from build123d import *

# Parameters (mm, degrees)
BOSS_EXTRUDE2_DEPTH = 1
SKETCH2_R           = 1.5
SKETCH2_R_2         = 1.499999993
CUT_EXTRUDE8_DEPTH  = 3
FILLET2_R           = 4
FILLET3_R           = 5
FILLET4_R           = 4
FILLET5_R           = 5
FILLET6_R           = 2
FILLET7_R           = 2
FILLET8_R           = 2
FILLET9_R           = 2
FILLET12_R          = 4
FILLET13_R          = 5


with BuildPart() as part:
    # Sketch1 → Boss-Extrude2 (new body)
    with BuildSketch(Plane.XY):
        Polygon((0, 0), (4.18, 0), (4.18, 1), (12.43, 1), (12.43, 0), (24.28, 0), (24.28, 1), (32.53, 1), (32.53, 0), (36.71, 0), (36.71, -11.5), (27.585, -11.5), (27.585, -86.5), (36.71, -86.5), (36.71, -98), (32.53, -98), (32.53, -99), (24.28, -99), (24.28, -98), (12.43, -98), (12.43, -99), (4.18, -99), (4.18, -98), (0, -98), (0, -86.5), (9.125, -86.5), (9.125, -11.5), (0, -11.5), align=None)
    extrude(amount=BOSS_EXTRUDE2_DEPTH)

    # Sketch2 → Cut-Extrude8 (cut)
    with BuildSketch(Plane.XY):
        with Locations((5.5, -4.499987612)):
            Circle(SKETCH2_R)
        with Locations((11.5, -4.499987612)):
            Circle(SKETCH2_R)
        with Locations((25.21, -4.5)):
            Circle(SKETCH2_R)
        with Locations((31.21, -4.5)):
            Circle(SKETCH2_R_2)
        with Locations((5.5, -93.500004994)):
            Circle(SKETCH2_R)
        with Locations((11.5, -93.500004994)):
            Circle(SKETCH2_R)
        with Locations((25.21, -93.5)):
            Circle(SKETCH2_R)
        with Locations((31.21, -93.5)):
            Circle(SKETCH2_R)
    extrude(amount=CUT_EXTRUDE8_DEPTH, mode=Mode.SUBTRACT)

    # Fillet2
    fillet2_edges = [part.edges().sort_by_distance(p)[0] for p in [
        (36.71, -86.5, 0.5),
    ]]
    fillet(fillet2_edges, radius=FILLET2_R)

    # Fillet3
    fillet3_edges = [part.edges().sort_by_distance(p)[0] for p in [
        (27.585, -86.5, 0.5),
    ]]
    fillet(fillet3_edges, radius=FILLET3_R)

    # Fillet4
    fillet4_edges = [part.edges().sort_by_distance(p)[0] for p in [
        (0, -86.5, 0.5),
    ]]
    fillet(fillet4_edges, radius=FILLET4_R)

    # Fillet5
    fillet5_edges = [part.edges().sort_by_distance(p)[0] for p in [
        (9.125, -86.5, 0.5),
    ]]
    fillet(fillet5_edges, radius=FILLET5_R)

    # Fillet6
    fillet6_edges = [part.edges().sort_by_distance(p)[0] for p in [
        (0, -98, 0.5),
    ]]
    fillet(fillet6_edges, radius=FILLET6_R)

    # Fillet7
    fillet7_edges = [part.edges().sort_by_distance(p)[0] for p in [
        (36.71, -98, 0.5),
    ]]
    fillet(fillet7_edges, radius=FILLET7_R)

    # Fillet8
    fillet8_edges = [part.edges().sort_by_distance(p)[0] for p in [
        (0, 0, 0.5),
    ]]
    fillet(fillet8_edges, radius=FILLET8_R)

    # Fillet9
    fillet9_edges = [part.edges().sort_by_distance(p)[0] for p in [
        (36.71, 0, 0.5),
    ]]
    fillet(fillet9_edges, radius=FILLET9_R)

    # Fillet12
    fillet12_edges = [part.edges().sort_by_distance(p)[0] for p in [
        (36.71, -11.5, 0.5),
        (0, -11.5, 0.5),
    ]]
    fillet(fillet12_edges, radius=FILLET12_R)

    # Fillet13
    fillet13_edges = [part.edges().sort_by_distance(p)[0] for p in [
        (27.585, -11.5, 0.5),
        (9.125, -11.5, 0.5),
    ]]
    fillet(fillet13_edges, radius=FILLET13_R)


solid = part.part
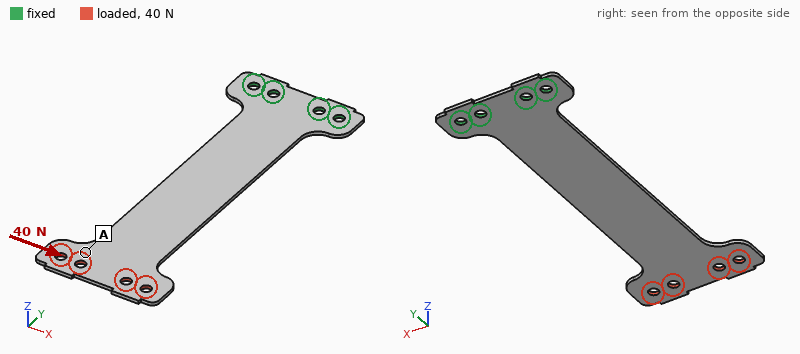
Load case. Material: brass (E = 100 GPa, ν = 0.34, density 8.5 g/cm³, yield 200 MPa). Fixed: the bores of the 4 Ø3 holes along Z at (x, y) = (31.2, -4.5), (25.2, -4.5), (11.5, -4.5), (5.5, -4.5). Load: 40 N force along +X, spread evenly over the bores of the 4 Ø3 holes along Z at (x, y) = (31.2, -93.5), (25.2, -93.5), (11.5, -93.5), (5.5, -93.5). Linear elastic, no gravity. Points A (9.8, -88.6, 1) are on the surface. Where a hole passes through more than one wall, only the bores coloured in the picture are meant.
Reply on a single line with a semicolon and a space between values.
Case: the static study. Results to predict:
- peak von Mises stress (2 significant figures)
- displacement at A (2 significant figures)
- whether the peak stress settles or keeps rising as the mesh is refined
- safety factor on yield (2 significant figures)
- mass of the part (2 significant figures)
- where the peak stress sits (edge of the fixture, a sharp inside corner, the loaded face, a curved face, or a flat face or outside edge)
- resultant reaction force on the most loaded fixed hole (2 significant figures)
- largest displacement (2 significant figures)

77 MPa; 0.14 mm; settles; 2.6; 19 g; a curved face; 110 N; 0.17 mm
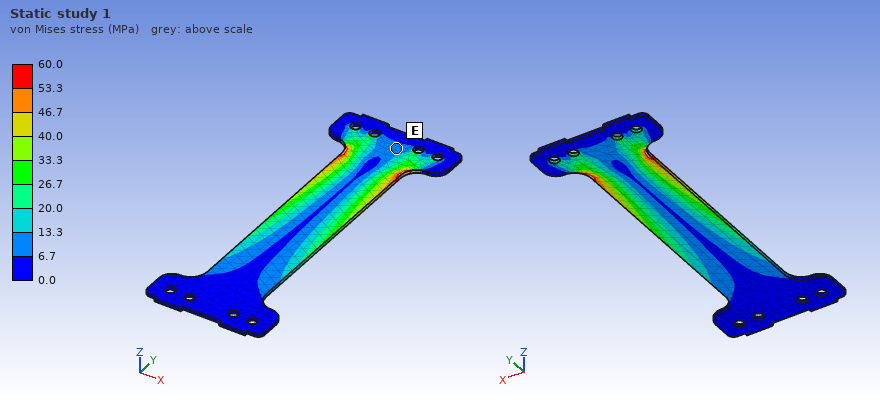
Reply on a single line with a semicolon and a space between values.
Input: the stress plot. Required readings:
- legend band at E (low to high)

6.7 to 13.3 MPa
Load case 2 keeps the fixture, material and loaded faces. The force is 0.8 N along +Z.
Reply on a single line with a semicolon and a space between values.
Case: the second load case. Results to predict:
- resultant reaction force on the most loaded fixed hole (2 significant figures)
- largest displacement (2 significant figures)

1.1 N; 1.2 mm
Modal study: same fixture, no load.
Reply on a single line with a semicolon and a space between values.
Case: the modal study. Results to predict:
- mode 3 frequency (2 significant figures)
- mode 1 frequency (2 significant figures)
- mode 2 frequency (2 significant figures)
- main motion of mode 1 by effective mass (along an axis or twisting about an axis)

390 Hz; 57 Hz; 390 Hz; along Z
